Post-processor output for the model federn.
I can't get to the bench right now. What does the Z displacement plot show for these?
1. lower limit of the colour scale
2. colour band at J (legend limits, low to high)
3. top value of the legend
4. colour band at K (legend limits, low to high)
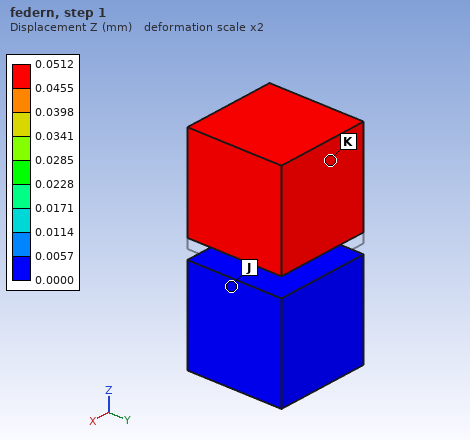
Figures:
0.0000 mm
0.0000 to 0.0057 mm
0.0512 mm
0.0455 to 0.0512 mm
